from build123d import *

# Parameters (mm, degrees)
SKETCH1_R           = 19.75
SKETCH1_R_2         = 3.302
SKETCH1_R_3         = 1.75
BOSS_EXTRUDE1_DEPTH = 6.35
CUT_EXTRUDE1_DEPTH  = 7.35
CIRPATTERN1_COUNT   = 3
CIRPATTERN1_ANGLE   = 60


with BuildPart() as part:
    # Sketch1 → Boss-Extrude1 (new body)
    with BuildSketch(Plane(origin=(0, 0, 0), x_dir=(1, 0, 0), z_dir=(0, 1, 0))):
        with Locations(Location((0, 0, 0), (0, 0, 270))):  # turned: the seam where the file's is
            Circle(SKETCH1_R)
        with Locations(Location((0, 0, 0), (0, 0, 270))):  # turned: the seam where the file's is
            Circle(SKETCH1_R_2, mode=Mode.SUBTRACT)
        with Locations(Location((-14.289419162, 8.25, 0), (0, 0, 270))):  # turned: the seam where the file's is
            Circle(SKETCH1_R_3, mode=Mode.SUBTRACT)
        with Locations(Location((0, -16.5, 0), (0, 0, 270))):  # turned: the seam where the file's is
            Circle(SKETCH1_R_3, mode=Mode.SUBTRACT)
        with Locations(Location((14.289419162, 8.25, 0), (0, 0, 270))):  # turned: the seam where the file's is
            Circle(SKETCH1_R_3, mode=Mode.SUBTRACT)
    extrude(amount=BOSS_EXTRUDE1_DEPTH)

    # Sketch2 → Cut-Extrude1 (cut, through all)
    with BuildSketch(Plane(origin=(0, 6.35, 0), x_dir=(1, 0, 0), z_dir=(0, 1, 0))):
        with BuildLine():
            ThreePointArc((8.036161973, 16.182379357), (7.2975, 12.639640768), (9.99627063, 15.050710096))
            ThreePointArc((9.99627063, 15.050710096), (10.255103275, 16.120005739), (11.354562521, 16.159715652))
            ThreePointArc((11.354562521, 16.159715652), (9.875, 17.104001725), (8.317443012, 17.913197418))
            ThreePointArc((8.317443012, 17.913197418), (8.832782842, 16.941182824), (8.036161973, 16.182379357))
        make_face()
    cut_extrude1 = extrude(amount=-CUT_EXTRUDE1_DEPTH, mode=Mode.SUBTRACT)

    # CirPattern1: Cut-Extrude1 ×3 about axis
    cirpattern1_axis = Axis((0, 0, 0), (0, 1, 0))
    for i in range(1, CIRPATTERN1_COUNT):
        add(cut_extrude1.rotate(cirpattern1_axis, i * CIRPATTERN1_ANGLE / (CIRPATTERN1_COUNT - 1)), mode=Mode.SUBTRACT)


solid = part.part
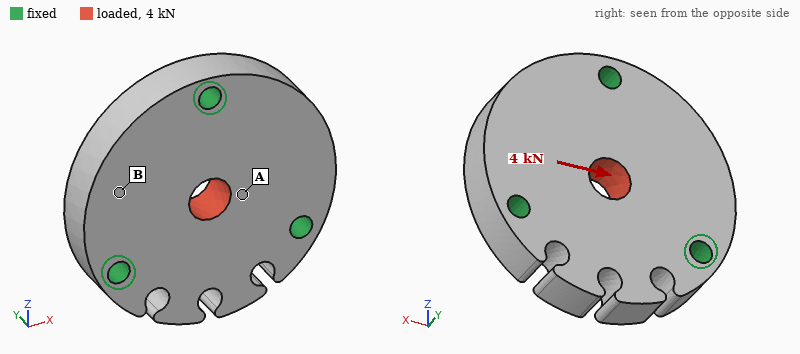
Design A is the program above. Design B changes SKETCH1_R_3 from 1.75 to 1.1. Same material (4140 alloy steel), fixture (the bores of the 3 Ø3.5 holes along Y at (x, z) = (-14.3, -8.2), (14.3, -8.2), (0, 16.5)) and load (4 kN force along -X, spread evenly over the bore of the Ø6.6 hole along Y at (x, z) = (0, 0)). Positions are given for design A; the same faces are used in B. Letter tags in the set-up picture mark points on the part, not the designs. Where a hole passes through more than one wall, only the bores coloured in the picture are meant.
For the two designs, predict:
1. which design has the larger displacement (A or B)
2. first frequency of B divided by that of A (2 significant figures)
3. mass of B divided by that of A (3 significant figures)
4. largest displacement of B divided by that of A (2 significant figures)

B
0.92
1.02
1.1
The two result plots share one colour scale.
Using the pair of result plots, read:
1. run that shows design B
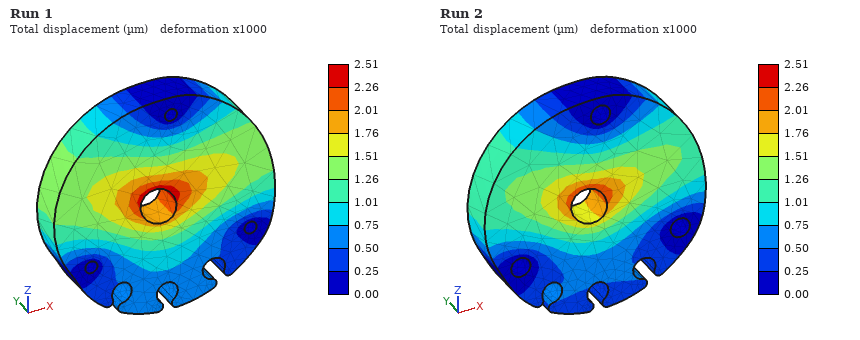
Run 1
